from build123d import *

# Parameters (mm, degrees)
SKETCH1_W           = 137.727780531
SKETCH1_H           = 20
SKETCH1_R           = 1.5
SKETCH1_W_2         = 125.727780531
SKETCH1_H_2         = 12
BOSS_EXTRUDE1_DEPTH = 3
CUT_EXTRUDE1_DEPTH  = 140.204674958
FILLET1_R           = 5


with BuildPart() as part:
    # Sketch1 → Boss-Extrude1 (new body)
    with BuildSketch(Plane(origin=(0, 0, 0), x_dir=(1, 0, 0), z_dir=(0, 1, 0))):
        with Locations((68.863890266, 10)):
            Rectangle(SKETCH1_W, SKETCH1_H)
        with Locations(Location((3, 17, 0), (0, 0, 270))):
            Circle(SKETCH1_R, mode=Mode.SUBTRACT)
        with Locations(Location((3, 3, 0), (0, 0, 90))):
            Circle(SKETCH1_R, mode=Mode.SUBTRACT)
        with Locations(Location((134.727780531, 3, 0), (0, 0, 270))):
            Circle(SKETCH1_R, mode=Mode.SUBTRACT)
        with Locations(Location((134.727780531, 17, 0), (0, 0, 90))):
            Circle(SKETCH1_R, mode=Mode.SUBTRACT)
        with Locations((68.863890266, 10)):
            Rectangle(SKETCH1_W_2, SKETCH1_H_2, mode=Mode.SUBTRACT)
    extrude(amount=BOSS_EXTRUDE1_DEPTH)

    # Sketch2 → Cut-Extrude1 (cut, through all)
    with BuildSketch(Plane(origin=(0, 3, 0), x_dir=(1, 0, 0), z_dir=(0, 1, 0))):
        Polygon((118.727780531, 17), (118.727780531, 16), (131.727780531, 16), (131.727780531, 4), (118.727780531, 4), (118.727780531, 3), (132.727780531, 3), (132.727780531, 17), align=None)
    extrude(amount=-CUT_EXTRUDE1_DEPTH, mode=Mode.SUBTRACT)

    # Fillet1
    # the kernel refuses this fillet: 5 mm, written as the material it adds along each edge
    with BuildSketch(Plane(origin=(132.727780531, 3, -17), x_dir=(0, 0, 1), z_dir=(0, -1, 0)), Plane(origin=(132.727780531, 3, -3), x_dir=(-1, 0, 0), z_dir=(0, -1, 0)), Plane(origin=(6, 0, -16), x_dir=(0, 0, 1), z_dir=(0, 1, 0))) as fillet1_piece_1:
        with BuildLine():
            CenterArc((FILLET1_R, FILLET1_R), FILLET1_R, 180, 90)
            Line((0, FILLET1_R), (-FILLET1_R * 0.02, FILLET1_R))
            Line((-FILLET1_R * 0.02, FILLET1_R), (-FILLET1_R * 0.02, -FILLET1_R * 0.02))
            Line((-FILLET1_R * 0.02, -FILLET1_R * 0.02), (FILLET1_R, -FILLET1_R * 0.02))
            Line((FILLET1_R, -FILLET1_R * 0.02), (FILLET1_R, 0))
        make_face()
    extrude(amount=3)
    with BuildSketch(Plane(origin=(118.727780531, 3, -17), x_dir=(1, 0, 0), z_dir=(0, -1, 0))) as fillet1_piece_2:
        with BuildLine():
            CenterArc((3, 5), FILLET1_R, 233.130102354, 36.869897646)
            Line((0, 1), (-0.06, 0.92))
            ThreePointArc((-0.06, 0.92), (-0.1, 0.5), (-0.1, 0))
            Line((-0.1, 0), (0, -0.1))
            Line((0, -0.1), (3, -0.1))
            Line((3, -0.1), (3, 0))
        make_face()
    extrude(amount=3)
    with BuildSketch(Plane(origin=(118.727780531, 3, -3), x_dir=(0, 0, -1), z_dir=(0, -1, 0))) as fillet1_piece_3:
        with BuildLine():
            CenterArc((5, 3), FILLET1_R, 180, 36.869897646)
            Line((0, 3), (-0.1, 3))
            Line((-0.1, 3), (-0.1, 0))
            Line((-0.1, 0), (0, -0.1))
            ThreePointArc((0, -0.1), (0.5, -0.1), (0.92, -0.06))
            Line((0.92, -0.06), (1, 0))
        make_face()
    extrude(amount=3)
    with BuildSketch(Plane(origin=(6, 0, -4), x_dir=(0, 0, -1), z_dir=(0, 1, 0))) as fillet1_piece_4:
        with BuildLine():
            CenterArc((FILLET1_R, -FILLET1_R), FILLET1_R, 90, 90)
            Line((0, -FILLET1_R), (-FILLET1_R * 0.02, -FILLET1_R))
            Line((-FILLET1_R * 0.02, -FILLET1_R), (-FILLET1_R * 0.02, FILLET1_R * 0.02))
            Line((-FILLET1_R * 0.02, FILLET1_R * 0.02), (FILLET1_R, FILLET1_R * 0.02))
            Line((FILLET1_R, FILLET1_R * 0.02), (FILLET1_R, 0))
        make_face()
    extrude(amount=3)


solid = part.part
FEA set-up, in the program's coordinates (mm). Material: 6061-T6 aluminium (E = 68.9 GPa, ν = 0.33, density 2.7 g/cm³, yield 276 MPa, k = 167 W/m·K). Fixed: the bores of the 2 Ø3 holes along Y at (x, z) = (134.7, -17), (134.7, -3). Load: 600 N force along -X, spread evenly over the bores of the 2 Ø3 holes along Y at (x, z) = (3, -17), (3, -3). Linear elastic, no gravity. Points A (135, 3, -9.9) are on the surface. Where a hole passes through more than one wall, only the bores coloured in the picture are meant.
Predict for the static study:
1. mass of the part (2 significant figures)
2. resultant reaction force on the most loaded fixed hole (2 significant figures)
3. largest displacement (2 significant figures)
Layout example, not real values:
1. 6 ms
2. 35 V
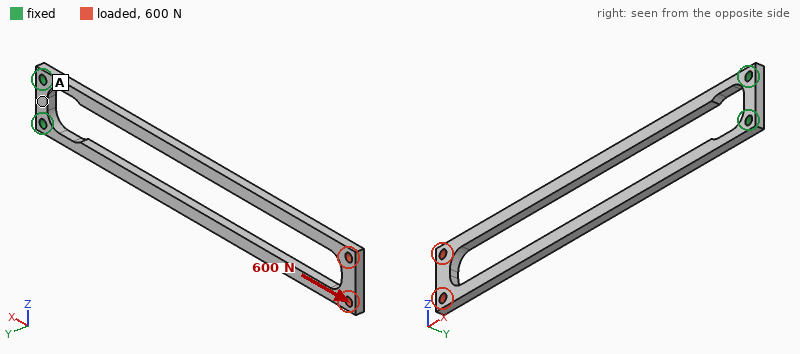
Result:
1. 9.7 g
2. 300 N
3. 52 µm
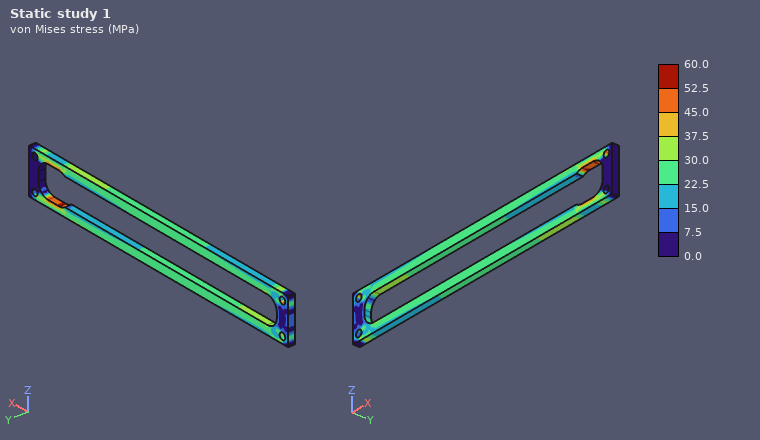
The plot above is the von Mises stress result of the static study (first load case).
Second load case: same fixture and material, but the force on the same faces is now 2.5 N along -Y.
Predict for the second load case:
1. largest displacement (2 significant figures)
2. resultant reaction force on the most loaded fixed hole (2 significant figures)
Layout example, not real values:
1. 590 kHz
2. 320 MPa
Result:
1. 1.7 mm
2. 1.3 N
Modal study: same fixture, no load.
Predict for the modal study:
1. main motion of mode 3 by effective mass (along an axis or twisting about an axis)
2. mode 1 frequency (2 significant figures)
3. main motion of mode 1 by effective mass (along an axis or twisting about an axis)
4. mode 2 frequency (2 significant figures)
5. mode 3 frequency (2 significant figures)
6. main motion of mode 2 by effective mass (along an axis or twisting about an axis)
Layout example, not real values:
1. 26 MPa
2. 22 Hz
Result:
1. twisting about X
2. 120 Hz
3. along Y
4. 250 Hz
5. 710 Hz
6. along Z
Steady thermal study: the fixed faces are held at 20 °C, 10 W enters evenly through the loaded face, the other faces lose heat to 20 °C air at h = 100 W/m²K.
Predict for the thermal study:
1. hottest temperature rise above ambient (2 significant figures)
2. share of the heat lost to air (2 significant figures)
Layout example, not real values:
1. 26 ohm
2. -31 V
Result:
1. 75 K
2. 95 %
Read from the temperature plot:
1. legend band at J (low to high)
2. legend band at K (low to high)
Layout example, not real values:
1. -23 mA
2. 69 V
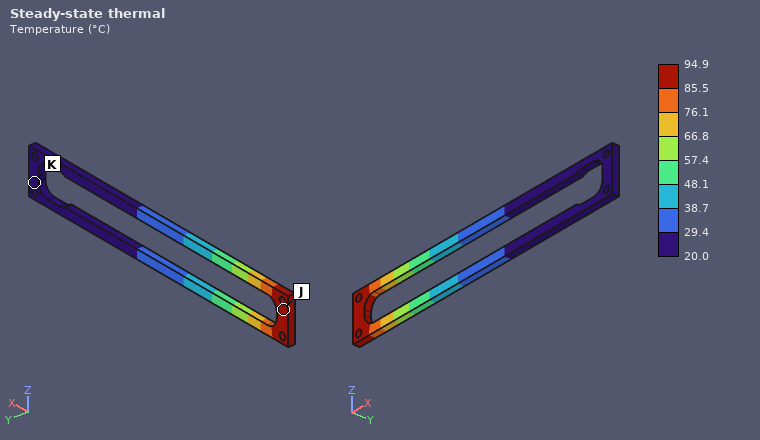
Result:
1. 85.5 to 94.9 °C
2. 20.0 to 29.4 °C
